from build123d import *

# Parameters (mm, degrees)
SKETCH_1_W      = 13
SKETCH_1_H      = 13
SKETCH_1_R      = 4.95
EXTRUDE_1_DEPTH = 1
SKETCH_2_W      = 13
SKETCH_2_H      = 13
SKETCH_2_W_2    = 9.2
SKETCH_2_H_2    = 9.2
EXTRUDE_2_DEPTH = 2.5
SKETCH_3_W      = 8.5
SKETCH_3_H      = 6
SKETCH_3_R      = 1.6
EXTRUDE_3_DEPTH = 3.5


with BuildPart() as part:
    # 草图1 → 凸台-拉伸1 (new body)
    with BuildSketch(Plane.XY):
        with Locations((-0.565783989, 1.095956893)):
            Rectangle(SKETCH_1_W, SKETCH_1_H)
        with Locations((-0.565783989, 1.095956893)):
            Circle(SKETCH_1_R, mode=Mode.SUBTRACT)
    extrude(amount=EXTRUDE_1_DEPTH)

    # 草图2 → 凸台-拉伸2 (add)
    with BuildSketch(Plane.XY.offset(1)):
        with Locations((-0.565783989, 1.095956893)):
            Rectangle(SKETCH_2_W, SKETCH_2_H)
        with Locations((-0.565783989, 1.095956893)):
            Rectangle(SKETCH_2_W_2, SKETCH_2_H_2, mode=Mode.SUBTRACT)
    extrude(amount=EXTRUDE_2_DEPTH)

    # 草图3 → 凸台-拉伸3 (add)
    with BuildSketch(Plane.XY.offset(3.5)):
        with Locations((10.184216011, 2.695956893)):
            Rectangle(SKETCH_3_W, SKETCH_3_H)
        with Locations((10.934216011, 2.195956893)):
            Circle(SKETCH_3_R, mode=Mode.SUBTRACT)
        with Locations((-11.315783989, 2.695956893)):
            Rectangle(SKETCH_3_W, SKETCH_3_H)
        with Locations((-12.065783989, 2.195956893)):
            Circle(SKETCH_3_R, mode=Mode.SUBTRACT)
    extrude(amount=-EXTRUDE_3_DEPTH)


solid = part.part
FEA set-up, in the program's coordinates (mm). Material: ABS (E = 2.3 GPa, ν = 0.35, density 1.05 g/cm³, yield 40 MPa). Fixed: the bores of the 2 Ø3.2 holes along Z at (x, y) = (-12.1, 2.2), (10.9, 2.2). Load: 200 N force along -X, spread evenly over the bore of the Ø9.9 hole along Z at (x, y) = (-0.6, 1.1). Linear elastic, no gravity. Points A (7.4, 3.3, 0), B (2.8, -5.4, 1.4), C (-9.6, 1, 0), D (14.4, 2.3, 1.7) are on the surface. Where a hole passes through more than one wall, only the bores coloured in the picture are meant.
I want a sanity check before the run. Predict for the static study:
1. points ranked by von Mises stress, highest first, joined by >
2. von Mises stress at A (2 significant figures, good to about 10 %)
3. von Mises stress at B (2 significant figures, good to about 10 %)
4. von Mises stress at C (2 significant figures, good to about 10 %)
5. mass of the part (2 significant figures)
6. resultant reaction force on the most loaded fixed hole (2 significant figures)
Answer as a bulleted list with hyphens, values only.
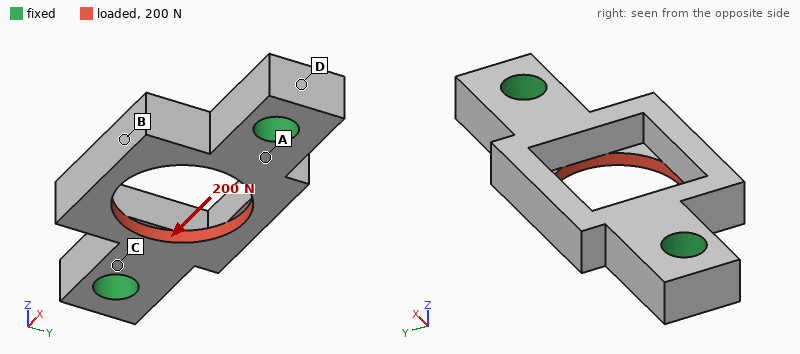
- B > C > A > D
- 5.1 MPa
- 14 MPa
- 9.9 MPa
- 0.63 g
- 100 N
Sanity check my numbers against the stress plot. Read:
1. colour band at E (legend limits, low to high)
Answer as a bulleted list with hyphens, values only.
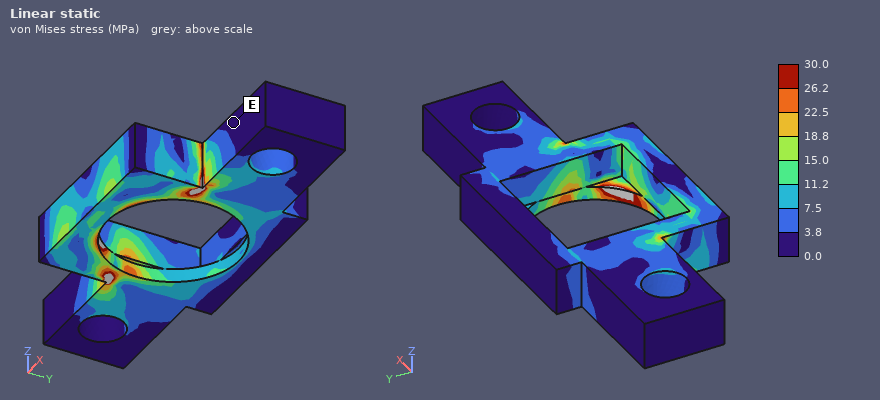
- 0.0 to 3.8 MPa
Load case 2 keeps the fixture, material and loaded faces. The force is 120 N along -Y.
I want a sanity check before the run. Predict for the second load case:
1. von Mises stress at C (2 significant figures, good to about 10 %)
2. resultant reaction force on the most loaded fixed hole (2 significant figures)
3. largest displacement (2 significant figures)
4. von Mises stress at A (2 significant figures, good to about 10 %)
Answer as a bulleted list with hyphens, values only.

- 12 MPa
- 62 N
- 0.13 mm
- 12 MPa
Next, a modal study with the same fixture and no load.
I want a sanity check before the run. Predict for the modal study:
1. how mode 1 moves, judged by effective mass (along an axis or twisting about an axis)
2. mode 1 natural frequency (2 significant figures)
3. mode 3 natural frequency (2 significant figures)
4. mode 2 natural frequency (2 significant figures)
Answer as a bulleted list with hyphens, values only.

- along Z
- 6300 Hz
- 11 kHz
- 10 kHz
